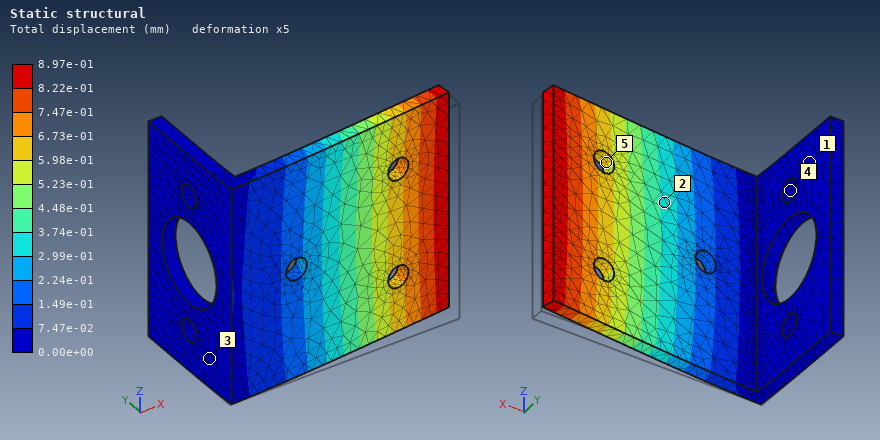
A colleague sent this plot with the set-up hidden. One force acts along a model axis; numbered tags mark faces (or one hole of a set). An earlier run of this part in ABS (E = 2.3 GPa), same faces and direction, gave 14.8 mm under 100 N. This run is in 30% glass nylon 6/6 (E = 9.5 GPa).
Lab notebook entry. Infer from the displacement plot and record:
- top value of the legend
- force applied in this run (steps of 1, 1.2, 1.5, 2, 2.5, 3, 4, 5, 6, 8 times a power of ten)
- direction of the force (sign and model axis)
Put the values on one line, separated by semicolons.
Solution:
8.97e-01 mm; 25 N; +Y
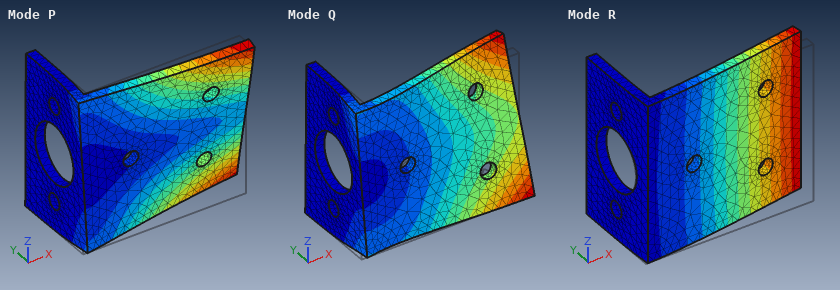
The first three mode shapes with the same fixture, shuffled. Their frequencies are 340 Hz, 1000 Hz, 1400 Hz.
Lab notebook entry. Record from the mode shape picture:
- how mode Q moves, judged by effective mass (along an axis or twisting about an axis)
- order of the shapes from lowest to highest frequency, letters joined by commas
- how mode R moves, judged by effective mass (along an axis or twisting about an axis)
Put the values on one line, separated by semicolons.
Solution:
along Z; R, P, Q; along Y
